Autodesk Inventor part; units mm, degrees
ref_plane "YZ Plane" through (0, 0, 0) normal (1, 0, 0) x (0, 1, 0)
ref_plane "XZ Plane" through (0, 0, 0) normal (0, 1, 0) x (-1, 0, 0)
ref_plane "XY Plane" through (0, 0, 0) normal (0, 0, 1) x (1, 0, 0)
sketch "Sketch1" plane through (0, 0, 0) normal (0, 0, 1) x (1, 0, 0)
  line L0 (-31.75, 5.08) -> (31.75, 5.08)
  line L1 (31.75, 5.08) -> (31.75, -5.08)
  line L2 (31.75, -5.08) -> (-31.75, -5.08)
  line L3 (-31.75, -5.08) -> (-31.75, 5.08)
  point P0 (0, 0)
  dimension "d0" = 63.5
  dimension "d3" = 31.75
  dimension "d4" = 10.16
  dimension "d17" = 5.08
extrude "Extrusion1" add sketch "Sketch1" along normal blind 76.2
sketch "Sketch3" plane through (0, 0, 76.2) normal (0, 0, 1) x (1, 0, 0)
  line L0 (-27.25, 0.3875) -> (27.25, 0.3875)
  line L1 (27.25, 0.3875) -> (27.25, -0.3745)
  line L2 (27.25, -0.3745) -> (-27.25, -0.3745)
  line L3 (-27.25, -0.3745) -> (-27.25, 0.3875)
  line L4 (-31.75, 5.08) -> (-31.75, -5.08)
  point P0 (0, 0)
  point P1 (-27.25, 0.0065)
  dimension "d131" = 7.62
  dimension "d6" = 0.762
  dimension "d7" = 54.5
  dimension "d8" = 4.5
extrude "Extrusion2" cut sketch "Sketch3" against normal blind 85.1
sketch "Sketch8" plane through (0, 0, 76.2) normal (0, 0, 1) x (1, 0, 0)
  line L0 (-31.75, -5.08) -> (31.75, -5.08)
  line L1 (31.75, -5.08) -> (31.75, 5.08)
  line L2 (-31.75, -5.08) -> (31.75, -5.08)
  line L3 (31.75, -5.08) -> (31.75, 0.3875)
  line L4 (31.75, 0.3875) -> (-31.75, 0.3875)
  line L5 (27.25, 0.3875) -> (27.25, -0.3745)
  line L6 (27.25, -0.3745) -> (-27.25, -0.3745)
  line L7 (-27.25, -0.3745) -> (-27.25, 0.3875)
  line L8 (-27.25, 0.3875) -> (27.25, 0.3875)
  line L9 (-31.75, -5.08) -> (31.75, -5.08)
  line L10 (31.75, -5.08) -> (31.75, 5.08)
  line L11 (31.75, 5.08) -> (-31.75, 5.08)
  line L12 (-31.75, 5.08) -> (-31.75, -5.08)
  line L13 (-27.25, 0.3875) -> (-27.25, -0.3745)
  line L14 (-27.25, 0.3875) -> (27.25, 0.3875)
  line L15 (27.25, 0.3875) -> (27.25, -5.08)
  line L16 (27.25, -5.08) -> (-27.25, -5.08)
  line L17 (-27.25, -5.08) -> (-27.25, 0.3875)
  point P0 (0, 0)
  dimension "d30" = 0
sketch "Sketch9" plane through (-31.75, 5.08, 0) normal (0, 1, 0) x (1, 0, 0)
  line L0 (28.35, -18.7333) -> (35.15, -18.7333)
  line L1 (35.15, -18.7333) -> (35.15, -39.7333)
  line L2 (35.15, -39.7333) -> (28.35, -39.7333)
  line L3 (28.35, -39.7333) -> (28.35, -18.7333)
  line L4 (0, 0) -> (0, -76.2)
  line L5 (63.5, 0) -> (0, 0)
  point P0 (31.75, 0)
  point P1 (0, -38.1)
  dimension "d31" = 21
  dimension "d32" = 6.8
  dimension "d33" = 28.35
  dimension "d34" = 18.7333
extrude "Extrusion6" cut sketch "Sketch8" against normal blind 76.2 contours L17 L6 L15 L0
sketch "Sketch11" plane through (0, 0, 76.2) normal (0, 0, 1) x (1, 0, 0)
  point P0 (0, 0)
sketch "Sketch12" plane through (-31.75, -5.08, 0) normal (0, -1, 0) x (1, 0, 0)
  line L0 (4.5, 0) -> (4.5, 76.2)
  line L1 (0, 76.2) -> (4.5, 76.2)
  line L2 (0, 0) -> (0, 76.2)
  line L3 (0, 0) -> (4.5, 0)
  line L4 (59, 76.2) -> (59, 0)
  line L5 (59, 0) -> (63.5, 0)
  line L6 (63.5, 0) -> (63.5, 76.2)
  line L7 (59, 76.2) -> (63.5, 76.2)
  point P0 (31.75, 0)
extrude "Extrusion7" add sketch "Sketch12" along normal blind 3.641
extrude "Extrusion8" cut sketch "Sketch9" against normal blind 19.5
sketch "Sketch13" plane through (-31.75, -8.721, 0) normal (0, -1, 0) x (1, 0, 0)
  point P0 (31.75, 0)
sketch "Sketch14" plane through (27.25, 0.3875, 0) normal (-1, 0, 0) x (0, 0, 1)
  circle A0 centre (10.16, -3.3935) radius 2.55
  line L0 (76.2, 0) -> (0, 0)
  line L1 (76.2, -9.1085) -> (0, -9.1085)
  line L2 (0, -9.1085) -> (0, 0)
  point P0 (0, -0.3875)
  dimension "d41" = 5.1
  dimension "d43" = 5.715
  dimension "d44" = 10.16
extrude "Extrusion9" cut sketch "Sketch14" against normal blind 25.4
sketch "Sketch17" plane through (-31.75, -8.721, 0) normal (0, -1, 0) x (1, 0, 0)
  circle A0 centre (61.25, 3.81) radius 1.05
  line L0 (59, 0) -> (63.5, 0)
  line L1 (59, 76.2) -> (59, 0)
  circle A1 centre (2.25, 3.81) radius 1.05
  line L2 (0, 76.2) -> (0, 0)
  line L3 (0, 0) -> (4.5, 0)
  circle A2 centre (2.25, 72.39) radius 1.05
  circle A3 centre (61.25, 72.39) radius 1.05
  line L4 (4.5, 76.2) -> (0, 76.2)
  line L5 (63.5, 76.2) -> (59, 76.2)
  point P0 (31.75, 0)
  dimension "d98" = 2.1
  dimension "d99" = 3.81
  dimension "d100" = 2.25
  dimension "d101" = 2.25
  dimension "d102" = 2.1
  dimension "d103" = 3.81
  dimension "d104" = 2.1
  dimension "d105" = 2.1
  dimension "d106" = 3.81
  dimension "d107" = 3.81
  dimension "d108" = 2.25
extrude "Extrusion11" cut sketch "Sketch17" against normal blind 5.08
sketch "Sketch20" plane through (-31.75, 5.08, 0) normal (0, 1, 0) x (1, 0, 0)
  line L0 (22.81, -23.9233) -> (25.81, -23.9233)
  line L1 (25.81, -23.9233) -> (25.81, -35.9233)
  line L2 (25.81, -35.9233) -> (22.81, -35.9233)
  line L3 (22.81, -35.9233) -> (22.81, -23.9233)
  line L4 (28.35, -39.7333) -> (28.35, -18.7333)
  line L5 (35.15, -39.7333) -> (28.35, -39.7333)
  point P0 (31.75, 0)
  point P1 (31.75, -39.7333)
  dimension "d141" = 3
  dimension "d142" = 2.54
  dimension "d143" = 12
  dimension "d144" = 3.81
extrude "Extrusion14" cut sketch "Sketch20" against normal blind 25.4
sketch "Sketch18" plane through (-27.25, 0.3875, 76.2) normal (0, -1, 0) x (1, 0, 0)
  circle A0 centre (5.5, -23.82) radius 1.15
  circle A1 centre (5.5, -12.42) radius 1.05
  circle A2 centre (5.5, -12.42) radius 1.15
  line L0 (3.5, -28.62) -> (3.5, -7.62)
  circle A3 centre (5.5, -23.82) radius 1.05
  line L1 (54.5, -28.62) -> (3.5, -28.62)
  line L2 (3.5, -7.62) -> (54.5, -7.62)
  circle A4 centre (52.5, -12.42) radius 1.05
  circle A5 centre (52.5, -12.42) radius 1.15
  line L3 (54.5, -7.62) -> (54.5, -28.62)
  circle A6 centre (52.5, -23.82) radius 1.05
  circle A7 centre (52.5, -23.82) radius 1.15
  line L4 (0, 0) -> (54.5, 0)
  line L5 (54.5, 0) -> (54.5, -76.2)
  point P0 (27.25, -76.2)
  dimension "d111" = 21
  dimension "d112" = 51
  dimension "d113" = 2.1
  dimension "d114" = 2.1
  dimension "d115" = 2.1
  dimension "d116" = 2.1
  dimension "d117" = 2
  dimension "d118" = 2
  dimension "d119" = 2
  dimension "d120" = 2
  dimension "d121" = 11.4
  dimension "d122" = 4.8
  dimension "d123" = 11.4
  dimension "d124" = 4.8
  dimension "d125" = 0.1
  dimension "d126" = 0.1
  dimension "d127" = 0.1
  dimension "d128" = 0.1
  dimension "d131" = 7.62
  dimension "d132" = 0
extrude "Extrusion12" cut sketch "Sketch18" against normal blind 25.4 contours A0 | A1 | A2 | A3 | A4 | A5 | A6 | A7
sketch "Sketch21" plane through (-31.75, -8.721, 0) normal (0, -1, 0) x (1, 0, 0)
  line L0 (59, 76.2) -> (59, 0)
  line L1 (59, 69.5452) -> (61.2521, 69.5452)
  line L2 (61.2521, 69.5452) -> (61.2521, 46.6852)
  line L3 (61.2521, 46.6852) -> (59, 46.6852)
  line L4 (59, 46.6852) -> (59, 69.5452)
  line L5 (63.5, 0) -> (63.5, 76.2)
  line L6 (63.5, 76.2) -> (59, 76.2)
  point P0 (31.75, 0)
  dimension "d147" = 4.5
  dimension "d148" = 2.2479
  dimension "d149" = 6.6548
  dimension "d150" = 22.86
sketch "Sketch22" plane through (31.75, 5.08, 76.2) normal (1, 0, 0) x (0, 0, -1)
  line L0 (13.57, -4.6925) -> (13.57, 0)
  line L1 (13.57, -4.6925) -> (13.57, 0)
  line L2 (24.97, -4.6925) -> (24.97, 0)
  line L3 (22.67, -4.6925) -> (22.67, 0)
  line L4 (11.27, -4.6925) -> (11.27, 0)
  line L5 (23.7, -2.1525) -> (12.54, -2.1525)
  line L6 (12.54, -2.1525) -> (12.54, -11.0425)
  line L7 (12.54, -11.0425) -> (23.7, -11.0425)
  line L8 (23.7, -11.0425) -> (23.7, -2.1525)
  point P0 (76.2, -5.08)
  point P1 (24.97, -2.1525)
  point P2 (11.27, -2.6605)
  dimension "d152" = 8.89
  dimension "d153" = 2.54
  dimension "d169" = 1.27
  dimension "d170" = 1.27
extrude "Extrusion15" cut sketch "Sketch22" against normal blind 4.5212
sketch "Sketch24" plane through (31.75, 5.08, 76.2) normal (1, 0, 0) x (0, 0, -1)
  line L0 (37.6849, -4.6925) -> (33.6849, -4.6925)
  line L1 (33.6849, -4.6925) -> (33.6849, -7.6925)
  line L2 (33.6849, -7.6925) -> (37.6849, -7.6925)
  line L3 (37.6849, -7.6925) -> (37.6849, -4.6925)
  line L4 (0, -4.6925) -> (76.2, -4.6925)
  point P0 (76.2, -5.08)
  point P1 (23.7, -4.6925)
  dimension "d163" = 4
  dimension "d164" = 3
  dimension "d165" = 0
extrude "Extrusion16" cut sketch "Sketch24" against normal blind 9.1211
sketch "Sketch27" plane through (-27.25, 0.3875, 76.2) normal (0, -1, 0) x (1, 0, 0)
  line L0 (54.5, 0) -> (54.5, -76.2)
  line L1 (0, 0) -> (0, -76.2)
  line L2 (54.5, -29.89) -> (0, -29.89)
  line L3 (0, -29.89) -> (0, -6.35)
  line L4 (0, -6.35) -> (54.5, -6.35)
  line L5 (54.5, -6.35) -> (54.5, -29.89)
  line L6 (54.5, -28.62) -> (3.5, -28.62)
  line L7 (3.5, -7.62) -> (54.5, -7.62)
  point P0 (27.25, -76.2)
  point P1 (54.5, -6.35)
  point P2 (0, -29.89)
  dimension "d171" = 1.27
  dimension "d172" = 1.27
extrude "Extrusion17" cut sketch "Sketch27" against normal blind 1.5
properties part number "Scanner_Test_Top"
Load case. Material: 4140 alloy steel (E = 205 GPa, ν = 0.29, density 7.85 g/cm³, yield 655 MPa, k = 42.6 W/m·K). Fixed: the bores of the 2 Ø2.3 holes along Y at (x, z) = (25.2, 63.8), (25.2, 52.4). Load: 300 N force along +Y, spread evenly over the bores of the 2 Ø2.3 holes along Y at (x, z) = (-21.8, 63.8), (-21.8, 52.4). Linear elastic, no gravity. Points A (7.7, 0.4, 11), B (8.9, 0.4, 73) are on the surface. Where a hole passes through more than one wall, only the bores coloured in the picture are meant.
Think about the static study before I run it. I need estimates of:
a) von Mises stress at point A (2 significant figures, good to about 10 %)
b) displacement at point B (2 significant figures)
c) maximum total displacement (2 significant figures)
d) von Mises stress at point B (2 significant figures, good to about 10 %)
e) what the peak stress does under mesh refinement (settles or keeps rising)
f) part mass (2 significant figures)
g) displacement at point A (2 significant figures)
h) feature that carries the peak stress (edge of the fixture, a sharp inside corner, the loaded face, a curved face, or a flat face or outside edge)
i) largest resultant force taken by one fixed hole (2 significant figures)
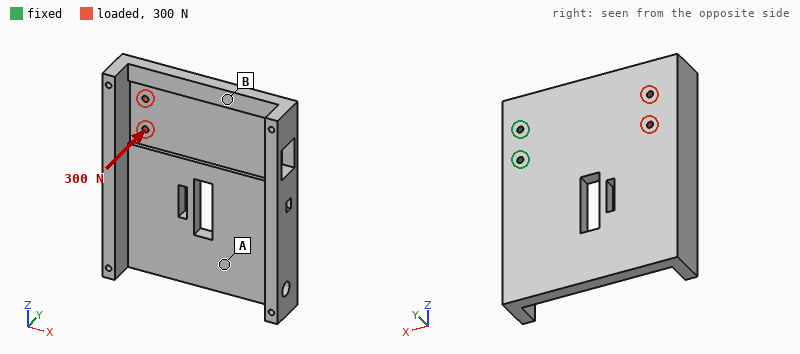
27 MPa
0.067 mm
0.37 mm
97 MPa
keeps rising
200 g
0.085 mm
edge of the fixture
210 N
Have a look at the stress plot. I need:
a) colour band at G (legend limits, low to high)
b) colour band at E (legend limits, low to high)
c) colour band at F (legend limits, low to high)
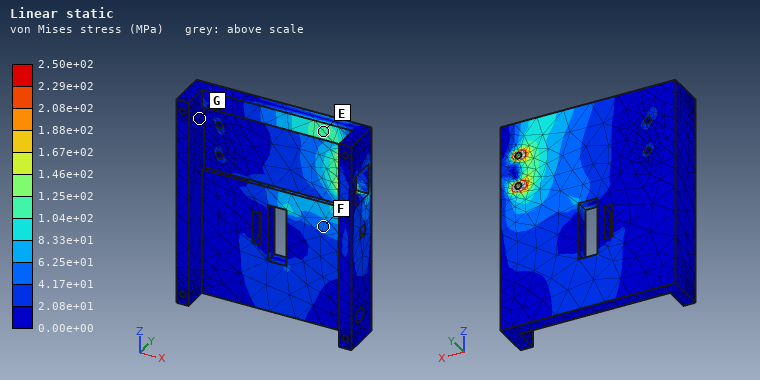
0.00e+00 to 2.08e+01 MPa
1.04e+02 to 1.25e+02 MPa
4.17e+01 to 6.25e+01 MPa
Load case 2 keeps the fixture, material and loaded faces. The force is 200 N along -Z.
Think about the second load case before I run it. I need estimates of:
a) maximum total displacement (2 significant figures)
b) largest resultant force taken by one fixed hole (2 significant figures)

16 µm
720 N
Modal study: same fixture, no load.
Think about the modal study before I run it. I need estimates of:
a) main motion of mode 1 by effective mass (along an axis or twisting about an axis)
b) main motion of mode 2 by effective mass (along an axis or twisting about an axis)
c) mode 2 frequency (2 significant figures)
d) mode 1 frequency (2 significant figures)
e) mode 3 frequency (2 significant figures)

along Y
twisting about X
1000 Hz
470 Hz
1700 Hz
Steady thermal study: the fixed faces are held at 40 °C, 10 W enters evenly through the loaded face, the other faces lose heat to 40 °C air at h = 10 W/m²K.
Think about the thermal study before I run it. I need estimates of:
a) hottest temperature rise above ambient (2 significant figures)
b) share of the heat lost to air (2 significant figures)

61 K
37 %
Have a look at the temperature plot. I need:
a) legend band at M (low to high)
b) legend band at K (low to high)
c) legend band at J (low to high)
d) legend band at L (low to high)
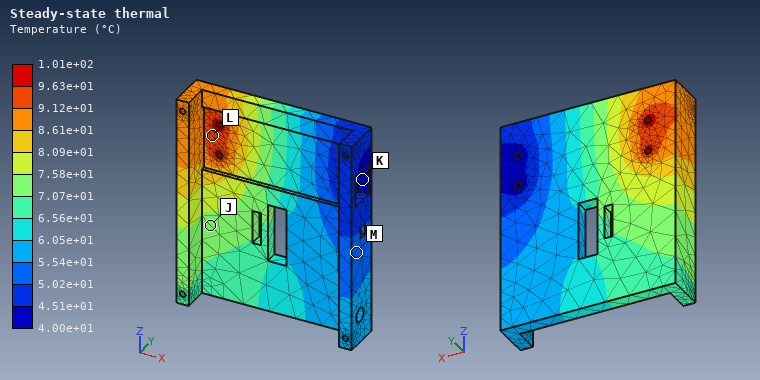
5.02e+01 to 5.54e+01 °C
4.00e+01 to 4.51e+01 °C
7.07e+01 to 7.58e+01 °C
9.12e+01 to 9.63e+01 °C
